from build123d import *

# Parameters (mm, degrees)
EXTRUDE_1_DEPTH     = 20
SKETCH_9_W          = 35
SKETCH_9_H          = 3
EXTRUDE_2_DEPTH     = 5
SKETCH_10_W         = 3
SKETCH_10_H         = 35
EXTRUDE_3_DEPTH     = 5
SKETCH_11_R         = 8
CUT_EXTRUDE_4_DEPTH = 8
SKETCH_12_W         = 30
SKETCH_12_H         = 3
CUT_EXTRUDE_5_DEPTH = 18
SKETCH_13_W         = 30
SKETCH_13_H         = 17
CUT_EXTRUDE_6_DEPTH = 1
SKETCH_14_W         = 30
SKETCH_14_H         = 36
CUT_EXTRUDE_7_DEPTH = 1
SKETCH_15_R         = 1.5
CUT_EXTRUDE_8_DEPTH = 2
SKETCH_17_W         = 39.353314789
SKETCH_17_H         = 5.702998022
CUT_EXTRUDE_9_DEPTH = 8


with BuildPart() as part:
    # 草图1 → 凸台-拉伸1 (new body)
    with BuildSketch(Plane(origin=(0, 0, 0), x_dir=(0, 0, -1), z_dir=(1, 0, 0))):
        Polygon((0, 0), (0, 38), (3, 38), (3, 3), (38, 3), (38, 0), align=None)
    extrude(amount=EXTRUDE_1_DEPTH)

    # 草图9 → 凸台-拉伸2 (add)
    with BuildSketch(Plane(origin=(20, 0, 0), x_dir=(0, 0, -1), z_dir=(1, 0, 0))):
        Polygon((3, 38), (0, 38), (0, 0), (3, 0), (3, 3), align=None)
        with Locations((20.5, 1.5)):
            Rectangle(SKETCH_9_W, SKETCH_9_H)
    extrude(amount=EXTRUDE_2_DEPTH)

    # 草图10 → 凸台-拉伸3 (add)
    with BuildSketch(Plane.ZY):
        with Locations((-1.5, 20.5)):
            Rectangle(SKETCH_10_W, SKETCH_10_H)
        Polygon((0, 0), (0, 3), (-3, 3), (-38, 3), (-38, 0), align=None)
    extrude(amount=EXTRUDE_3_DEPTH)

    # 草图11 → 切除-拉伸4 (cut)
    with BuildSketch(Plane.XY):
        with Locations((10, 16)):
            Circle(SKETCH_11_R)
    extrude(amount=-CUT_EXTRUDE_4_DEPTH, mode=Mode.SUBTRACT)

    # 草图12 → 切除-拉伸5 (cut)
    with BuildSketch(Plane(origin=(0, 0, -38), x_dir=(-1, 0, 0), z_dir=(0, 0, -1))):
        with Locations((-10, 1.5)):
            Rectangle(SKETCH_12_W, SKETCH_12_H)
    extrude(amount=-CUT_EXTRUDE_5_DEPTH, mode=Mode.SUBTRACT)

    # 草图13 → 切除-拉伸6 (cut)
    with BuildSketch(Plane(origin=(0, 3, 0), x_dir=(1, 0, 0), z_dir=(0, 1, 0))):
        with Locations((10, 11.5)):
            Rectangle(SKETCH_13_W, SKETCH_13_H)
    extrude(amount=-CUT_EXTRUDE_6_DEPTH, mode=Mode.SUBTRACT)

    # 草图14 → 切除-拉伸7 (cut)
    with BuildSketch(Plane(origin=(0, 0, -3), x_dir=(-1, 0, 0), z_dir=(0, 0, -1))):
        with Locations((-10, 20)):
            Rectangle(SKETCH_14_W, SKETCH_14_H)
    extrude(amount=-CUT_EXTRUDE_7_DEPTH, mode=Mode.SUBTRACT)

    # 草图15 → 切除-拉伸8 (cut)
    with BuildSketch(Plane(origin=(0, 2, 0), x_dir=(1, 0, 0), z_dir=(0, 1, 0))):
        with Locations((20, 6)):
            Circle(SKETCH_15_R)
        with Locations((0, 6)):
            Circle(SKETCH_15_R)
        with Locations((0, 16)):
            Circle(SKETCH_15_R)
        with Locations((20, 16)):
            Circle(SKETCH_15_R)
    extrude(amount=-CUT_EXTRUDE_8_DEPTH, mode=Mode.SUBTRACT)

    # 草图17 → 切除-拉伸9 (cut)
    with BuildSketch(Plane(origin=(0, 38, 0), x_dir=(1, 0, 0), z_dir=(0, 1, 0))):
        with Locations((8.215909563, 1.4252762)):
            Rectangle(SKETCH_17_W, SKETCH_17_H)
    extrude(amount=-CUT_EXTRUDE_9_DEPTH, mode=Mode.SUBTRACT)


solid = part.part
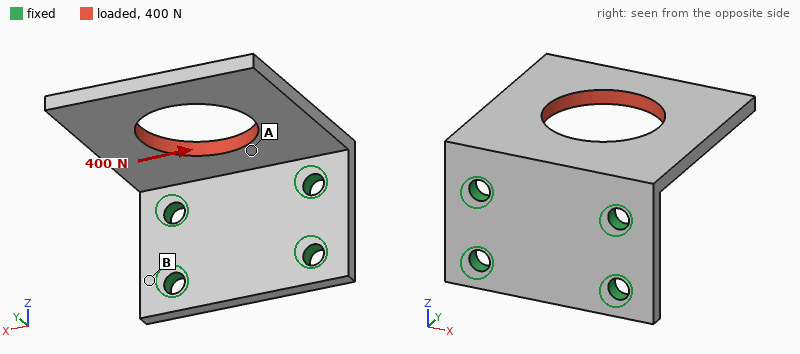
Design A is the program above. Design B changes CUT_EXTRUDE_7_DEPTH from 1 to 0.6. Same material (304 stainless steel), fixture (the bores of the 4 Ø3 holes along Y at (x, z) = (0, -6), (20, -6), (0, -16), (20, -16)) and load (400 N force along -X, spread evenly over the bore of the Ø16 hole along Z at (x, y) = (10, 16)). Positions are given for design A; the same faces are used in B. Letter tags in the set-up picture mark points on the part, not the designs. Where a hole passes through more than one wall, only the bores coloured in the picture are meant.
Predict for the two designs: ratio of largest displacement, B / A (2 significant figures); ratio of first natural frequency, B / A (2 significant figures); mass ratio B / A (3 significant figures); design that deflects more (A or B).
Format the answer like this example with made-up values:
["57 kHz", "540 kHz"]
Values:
["0.80", "1.1", "1.11", "A"]
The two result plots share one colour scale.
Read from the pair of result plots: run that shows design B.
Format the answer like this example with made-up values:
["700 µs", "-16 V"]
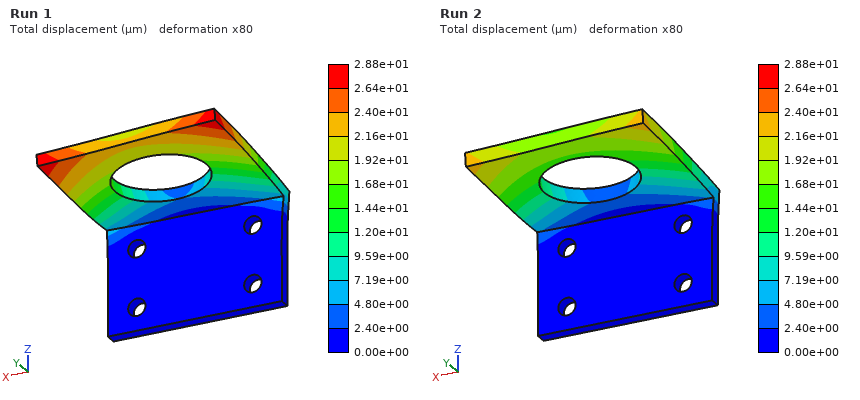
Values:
["Run 2"]
